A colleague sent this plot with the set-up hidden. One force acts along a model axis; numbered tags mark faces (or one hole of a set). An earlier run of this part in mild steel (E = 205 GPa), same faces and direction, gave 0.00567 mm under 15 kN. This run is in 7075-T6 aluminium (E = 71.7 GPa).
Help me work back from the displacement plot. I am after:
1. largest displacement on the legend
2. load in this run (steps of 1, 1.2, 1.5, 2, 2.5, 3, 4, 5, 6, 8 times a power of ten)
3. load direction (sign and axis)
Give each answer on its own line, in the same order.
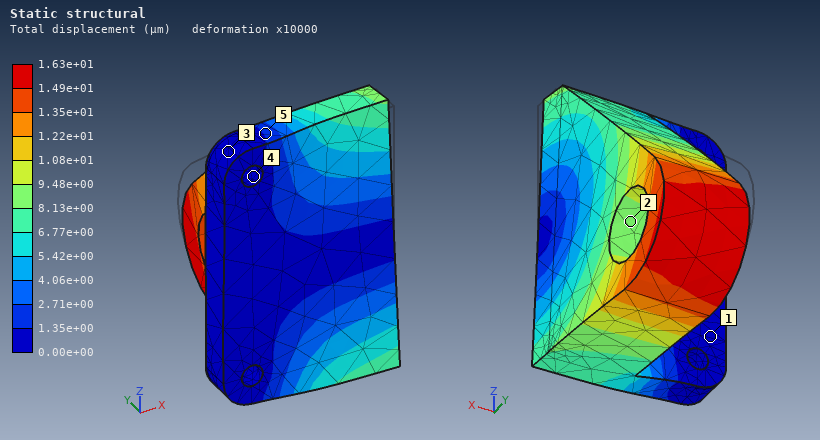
1.63e+01 µm
15 kN
-Z
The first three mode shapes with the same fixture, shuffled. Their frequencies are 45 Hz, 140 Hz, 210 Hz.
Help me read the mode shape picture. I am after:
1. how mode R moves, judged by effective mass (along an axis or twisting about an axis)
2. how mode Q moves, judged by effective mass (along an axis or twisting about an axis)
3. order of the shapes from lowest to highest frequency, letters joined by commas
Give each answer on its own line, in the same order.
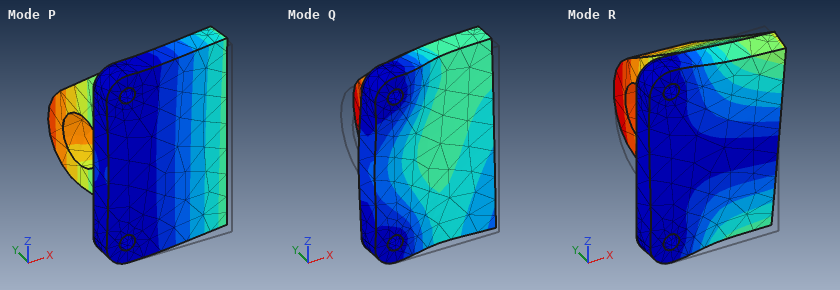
along Z
along Y
P, R, Q
